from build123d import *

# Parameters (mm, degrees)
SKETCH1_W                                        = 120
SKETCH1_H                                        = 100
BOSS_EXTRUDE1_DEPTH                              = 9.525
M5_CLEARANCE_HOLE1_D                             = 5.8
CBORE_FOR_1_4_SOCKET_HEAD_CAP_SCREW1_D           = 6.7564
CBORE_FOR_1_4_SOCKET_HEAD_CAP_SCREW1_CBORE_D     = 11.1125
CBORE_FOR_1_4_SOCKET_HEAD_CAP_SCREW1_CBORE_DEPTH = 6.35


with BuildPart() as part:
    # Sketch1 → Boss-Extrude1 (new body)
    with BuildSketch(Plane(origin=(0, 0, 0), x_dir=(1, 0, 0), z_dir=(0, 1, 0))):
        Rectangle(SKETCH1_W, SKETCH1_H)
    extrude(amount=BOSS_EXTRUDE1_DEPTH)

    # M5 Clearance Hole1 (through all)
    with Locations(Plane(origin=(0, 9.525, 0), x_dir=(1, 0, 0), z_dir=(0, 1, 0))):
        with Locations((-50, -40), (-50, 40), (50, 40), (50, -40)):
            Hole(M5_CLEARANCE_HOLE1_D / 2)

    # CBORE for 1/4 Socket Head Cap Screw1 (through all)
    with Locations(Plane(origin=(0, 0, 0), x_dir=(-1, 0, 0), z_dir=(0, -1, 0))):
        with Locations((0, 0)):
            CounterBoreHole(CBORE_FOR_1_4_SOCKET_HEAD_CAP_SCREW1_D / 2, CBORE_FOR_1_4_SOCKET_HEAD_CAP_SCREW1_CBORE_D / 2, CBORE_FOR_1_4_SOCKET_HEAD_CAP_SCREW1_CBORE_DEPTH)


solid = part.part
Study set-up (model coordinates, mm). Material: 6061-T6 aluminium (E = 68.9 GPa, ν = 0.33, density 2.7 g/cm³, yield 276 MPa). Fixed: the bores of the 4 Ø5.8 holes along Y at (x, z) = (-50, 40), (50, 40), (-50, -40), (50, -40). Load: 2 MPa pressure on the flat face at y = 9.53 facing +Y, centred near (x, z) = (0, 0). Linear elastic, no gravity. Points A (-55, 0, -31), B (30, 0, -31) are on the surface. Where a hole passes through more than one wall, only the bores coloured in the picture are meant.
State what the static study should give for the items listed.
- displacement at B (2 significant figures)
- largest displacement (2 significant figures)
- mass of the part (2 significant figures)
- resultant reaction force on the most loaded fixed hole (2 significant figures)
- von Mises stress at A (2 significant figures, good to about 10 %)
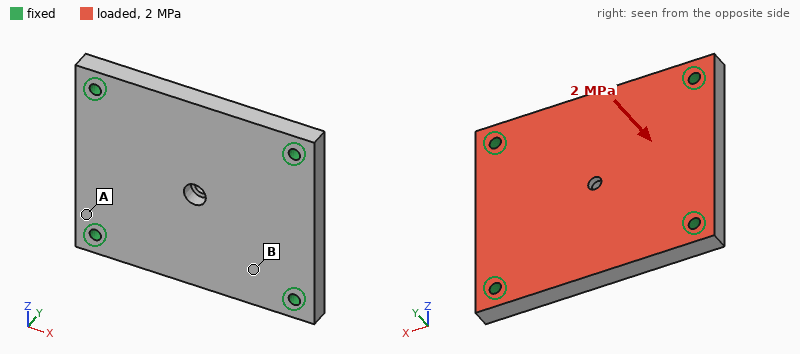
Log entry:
0.11 mm
0.23 mm
300 g
5.9 kN
60 MPa
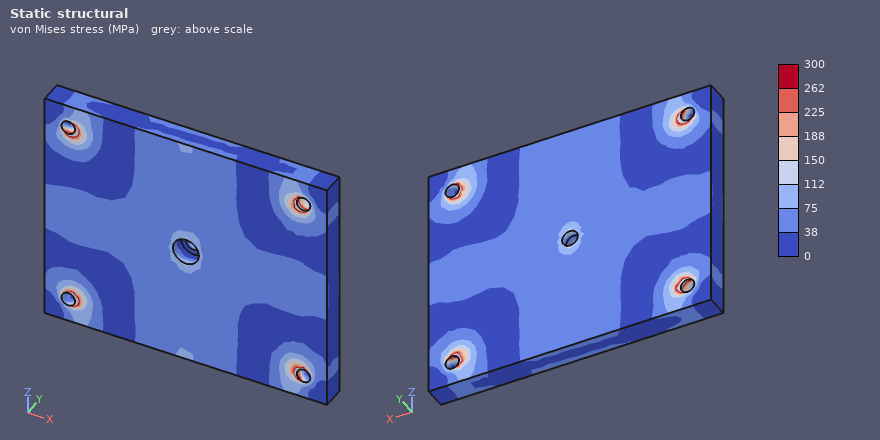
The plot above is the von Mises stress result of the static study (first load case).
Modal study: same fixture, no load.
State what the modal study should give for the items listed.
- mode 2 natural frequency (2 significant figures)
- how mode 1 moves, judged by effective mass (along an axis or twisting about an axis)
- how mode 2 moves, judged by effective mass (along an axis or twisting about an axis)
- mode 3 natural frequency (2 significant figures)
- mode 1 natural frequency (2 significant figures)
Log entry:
5400 Hz
along Y
twisting about X
6800 Hz
3600 Hz
